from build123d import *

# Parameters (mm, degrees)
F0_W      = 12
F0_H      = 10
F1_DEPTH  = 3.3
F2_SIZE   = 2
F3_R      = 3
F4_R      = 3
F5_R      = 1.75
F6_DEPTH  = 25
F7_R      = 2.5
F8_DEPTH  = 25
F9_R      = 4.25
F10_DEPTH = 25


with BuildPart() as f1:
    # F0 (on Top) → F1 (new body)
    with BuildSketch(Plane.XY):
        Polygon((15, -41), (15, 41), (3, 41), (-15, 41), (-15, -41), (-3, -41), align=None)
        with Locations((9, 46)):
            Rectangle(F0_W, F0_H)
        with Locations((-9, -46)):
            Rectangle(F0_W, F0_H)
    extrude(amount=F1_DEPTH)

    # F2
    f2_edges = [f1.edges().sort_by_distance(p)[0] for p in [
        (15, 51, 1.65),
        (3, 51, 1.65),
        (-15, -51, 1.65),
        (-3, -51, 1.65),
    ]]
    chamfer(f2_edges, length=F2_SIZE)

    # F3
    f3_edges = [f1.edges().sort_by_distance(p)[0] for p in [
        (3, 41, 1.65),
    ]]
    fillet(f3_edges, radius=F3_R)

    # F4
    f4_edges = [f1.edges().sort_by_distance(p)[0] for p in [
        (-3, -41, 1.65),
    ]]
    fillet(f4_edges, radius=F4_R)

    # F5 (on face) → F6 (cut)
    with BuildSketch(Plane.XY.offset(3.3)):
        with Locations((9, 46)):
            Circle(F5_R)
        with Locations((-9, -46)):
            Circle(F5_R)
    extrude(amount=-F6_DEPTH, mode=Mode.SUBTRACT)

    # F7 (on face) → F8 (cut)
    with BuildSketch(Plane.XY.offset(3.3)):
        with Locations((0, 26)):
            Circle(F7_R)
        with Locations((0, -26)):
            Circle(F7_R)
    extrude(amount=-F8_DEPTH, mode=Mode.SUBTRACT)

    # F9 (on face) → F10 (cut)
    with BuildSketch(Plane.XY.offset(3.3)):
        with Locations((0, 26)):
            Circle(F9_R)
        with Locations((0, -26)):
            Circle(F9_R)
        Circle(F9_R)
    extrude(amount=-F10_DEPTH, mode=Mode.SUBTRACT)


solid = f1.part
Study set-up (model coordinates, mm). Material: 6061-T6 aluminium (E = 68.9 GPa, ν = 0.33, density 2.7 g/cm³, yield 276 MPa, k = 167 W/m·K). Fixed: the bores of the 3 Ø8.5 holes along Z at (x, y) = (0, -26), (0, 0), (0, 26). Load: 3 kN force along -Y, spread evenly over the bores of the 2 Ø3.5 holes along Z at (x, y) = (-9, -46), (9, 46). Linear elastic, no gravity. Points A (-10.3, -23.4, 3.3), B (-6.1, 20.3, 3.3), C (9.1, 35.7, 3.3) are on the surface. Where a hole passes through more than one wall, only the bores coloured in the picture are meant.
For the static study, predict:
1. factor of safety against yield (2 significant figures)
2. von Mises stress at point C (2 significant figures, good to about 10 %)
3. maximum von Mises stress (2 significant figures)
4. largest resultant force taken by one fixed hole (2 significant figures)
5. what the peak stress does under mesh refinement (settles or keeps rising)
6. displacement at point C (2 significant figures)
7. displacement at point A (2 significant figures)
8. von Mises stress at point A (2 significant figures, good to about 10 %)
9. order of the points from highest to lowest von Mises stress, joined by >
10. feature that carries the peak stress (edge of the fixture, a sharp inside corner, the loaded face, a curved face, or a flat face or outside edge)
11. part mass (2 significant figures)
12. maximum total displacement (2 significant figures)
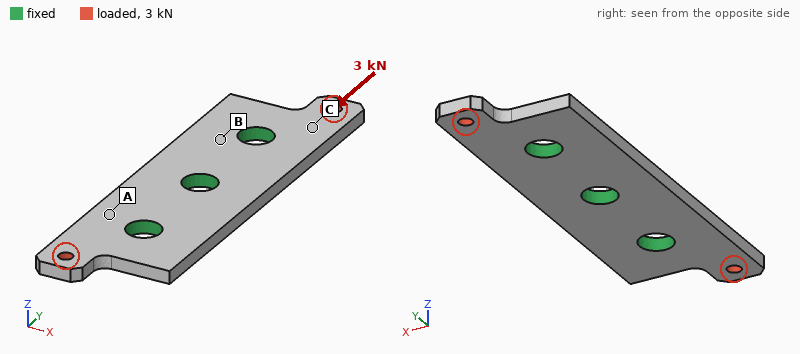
2.5
36 MPa
110 MPa
1.3 kN
settles
9.3 µm
4.0 µm
23 MPa
C > A > B
the loaded face
22 g
24 µm
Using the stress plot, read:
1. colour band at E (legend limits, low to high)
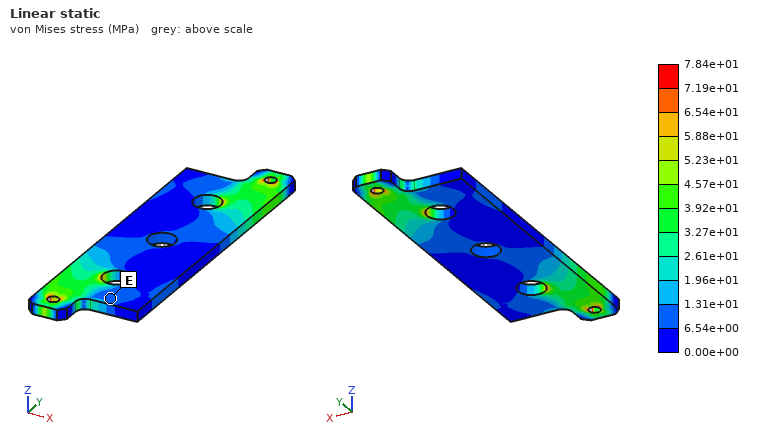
6.54e+00 to 1.31e+01 MPa
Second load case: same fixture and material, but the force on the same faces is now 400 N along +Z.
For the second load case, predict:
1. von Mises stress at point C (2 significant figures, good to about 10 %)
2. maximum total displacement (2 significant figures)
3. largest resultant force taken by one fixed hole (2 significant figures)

56 MPa
0.17 mm
220 N
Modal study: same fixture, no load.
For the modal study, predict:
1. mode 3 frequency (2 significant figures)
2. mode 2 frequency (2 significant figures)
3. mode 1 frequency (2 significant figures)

13 kHz
6300 Hz
6300 Hz
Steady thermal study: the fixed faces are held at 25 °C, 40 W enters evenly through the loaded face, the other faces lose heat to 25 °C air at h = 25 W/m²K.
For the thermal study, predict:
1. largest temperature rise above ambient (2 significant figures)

51 K
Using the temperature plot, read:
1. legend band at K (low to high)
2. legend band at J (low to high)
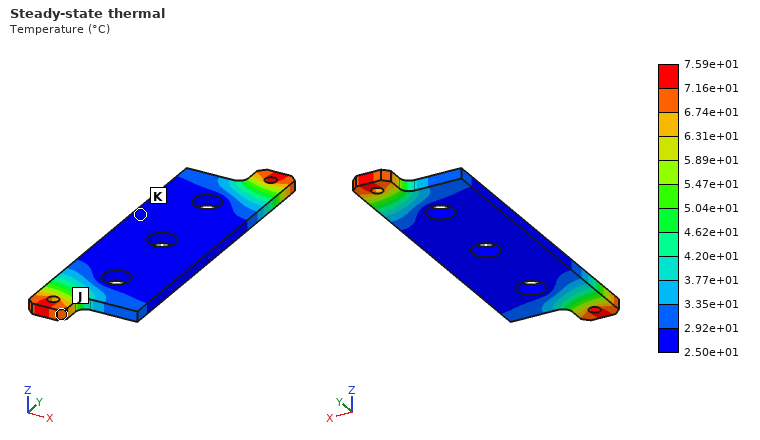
2.50e+01 to 2.92e+01 °C
6.74e+01 to 7.16e+01 °C
